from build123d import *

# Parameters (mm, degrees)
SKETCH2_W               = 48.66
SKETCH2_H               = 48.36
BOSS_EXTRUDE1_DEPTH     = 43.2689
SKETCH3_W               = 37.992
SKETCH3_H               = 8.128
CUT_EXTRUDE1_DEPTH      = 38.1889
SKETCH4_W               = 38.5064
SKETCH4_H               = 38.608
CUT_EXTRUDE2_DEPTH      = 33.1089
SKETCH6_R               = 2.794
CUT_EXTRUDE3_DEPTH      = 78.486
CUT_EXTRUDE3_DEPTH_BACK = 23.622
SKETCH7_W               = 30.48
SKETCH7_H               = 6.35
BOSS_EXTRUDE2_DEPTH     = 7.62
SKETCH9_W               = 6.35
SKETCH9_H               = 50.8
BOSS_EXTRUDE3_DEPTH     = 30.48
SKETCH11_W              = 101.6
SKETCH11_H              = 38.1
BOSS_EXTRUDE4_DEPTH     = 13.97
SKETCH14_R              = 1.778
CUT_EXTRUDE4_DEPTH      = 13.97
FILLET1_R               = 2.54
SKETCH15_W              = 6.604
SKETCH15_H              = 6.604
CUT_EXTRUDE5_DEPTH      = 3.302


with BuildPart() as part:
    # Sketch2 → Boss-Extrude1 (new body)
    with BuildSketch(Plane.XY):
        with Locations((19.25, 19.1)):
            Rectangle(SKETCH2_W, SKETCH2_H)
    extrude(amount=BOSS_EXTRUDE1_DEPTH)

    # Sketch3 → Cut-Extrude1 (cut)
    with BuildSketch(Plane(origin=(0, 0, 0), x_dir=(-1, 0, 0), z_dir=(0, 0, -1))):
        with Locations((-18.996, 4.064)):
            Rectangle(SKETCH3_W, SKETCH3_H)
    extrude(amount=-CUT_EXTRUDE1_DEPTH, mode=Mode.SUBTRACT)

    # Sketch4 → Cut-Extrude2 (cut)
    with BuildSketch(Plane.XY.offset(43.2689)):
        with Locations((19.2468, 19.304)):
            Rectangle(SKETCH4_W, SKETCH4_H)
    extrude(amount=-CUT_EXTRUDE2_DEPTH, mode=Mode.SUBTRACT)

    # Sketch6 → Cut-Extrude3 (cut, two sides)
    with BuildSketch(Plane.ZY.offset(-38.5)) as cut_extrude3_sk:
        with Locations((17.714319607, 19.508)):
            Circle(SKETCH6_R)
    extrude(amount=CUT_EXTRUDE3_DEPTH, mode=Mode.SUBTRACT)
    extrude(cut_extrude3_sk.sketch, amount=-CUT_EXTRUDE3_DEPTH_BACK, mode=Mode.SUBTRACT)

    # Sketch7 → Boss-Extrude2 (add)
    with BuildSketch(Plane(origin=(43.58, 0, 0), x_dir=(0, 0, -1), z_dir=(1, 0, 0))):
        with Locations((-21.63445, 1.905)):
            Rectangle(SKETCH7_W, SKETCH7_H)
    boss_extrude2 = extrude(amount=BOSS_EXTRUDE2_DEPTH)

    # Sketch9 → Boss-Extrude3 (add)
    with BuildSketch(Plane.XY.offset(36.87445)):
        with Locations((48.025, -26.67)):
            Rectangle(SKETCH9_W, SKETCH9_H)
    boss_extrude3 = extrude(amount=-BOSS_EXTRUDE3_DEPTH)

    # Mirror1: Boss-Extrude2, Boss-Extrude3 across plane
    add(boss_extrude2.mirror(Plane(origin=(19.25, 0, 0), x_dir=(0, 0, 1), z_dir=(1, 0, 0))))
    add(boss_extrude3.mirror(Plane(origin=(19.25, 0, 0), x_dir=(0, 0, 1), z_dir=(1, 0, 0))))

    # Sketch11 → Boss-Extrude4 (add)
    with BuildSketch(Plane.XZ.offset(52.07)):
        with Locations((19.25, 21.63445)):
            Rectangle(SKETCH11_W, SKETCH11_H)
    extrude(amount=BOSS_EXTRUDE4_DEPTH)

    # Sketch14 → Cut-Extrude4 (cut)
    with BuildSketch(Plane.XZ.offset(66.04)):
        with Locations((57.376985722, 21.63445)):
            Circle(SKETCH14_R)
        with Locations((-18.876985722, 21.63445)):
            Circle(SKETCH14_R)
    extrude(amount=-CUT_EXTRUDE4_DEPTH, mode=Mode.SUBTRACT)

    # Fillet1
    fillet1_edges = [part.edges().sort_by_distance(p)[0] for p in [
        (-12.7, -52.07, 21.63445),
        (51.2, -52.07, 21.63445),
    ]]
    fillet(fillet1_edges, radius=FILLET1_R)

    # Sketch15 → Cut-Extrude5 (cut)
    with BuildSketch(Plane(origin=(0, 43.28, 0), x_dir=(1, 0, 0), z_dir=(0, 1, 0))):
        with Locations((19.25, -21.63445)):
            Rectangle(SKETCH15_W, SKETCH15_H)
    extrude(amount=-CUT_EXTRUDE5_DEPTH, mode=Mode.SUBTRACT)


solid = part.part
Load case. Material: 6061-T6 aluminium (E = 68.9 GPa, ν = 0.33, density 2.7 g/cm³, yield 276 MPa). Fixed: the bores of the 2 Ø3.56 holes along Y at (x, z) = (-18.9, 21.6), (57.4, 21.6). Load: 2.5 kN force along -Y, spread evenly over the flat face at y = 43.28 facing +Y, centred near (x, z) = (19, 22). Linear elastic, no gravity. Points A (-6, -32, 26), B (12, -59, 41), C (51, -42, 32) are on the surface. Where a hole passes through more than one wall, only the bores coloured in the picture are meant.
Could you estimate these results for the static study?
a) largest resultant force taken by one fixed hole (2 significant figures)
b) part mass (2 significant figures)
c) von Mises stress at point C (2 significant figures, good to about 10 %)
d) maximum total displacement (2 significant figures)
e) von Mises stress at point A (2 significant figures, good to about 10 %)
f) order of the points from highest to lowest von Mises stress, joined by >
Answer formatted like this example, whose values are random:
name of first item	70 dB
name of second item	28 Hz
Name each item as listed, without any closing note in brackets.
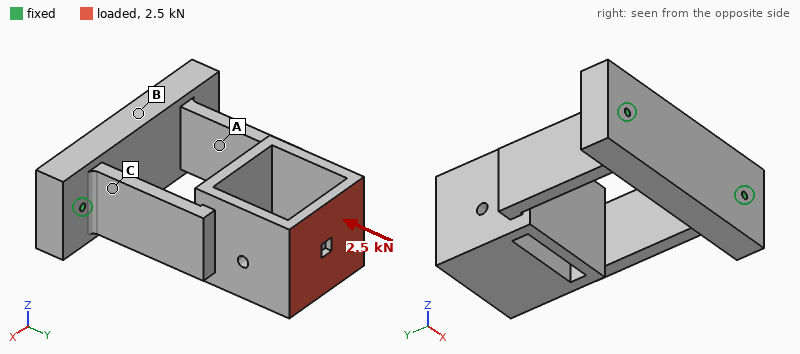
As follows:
largest resultant force taken by one fixed hole	1.3 kN
part mass	340 g
von Mises stress at point C	10 MPa
maximum total displacement	46 µm
von Mises stress at point A	6.3 MPa
order of the points from highest to lowest von Mises stress, joined by >	C > A > B
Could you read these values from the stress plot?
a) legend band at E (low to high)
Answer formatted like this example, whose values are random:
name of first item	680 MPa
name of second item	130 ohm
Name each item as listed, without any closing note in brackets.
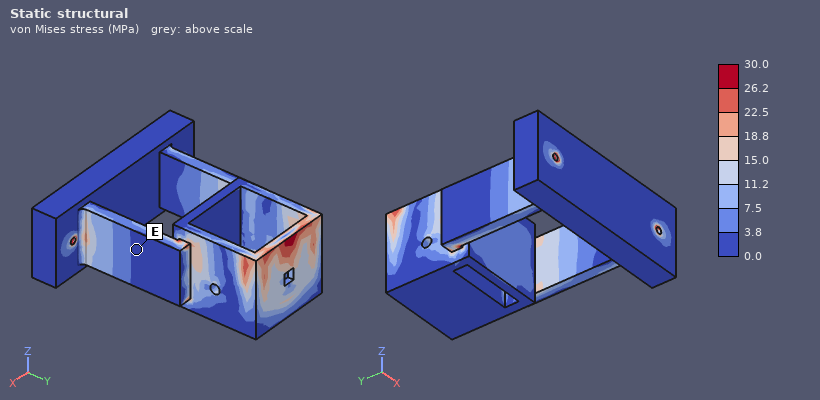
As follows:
legend band at E	0.0 to 3.8 MPa
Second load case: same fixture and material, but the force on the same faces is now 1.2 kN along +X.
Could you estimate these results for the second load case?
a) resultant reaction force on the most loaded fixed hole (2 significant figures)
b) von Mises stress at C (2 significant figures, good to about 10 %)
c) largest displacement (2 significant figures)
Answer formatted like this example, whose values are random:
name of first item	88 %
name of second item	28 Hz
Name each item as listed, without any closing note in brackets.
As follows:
resultant reaction force on the most loaded fixed hole	1.7 kN
von Mises stress at C	55 MPa
largest displacement	0.34 mm
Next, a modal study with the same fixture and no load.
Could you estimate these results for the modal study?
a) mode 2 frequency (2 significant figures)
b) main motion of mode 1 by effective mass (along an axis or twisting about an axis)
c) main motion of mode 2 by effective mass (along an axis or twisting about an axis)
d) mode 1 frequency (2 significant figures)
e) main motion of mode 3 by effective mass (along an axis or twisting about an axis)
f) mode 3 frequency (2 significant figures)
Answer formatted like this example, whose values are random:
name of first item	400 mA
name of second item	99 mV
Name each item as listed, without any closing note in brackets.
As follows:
mode 2 frequency	1000 Hz
main motion of mode 1 by effective mass	along X
main motion of mode 2 by effective mass	along Z
mode 1 frequency	880 Hz
main motion of mode 3 by effective mass	twisting about Y
mode 3 frequency	2300 Hz
